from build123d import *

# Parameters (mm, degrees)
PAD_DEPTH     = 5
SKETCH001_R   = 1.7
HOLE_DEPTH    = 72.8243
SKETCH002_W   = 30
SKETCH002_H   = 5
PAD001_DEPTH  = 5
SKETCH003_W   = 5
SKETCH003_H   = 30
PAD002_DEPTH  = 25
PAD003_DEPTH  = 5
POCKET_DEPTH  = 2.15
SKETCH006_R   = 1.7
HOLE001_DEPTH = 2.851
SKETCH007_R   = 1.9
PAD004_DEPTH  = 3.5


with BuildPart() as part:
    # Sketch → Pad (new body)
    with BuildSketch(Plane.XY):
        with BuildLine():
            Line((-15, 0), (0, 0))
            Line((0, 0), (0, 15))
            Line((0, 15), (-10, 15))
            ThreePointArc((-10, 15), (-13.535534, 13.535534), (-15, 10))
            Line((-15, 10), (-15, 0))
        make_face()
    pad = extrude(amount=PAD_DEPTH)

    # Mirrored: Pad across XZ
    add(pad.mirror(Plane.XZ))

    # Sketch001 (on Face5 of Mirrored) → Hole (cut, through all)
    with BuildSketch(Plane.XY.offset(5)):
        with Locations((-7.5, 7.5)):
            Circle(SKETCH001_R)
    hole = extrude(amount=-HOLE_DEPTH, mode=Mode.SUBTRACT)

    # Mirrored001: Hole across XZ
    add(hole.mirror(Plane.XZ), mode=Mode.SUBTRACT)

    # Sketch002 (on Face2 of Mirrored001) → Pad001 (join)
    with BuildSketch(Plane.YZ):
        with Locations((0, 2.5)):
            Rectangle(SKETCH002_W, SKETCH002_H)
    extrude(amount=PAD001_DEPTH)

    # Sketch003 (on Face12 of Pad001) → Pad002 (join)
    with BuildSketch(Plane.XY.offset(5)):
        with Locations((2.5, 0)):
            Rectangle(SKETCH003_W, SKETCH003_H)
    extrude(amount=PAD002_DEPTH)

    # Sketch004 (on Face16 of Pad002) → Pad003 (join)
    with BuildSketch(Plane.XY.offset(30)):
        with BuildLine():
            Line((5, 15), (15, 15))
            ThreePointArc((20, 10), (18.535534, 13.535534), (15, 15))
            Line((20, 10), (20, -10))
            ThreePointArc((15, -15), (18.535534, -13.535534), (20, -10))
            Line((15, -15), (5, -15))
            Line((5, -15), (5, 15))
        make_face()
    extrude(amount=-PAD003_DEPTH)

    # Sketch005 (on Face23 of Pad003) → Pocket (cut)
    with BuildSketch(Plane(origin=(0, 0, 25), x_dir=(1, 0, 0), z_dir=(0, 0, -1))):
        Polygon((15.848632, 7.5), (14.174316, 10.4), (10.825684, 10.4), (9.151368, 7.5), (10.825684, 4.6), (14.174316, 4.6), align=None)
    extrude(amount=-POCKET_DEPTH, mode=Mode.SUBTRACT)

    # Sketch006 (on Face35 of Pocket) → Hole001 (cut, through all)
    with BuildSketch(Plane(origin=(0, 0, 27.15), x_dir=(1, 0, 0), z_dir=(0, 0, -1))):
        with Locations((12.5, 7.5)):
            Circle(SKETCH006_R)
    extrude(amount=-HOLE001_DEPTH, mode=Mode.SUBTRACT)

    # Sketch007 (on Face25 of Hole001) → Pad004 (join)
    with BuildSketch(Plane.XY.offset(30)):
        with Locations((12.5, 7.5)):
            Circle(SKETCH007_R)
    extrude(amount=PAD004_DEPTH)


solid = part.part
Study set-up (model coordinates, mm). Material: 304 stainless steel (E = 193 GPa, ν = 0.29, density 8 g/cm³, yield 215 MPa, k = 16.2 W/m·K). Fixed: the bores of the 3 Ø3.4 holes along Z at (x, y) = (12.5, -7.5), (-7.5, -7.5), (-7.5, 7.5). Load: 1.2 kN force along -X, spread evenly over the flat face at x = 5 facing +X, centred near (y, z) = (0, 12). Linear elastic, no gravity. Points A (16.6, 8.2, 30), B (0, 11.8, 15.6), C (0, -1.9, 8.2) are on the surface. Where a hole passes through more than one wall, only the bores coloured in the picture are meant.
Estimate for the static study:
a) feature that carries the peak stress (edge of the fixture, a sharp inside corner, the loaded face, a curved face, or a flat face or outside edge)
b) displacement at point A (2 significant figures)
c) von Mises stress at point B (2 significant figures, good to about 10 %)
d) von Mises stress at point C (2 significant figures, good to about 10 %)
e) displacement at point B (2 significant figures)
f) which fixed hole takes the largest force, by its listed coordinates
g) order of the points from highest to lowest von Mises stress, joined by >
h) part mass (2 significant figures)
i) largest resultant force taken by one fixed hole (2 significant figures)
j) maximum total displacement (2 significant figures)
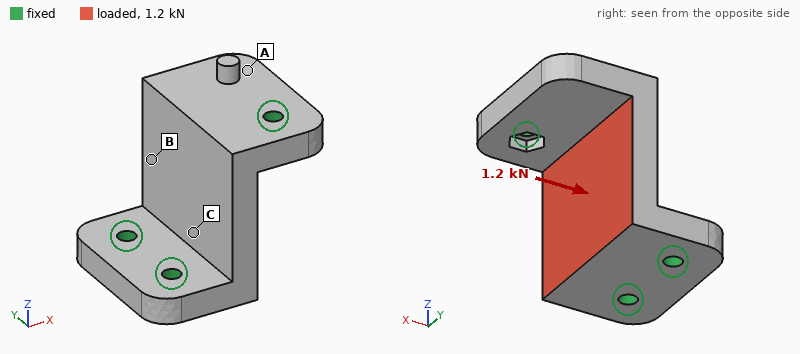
edge of the fixture
3.5 µm
21 MPa
11 MPa
5.9 µm
(12.5, -7.5)
B > C > A
70 g
460 N
7.3 µm
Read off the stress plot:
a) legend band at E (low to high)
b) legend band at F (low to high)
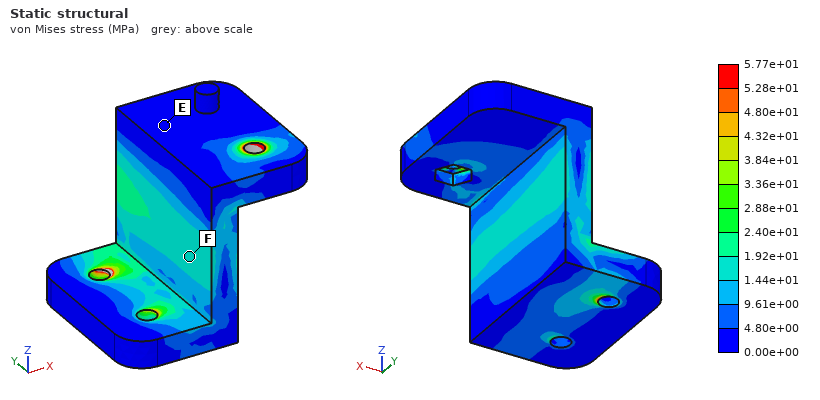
0.00e+00 to 4.80e+00 MPa
1.44e+01 to 1.92e+01 MPa
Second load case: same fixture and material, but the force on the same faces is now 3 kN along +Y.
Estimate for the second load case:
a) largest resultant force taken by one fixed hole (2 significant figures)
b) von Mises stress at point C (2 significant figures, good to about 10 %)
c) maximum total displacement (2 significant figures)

1.6 kN
28 MPa
13 µm
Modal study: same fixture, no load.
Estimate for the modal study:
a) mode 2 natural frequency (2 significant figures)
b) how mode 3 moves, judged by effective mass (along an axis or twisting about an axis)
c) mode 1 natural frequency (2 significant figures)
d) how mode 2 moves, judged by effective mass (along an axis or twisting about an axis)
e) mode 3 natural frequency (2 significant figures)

13 kHz
along Z
7600 Hz
along Z
15 kHz
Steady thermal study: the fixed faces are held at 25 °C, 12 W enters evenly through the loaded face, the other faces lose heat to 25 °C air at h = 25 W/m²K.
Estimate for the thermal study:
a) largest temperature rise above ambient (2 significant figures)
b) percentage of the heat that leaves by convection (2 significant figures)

42 K
15 %
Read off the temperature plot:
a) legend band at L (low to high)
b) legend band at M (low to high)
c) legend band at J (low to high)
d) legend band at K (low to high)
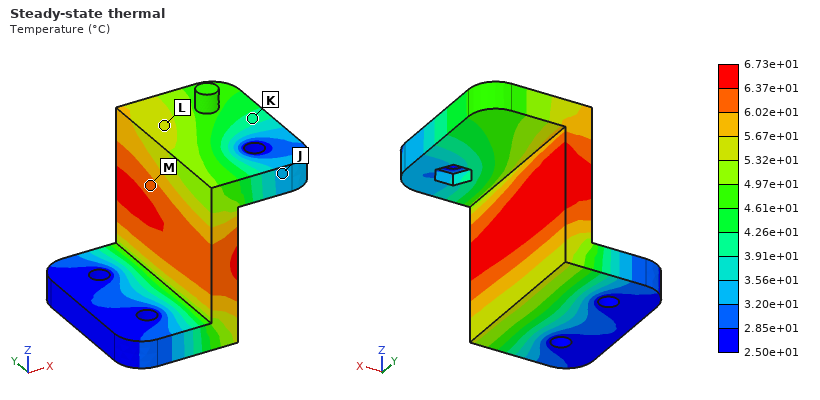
5.32e+01 to 5.67e+01 °C
6.02e+01 to 6.37e+01 °C
3.20e+01 to 3.56e+01 °C
3.91e+01 to 4.26e+01 °C
